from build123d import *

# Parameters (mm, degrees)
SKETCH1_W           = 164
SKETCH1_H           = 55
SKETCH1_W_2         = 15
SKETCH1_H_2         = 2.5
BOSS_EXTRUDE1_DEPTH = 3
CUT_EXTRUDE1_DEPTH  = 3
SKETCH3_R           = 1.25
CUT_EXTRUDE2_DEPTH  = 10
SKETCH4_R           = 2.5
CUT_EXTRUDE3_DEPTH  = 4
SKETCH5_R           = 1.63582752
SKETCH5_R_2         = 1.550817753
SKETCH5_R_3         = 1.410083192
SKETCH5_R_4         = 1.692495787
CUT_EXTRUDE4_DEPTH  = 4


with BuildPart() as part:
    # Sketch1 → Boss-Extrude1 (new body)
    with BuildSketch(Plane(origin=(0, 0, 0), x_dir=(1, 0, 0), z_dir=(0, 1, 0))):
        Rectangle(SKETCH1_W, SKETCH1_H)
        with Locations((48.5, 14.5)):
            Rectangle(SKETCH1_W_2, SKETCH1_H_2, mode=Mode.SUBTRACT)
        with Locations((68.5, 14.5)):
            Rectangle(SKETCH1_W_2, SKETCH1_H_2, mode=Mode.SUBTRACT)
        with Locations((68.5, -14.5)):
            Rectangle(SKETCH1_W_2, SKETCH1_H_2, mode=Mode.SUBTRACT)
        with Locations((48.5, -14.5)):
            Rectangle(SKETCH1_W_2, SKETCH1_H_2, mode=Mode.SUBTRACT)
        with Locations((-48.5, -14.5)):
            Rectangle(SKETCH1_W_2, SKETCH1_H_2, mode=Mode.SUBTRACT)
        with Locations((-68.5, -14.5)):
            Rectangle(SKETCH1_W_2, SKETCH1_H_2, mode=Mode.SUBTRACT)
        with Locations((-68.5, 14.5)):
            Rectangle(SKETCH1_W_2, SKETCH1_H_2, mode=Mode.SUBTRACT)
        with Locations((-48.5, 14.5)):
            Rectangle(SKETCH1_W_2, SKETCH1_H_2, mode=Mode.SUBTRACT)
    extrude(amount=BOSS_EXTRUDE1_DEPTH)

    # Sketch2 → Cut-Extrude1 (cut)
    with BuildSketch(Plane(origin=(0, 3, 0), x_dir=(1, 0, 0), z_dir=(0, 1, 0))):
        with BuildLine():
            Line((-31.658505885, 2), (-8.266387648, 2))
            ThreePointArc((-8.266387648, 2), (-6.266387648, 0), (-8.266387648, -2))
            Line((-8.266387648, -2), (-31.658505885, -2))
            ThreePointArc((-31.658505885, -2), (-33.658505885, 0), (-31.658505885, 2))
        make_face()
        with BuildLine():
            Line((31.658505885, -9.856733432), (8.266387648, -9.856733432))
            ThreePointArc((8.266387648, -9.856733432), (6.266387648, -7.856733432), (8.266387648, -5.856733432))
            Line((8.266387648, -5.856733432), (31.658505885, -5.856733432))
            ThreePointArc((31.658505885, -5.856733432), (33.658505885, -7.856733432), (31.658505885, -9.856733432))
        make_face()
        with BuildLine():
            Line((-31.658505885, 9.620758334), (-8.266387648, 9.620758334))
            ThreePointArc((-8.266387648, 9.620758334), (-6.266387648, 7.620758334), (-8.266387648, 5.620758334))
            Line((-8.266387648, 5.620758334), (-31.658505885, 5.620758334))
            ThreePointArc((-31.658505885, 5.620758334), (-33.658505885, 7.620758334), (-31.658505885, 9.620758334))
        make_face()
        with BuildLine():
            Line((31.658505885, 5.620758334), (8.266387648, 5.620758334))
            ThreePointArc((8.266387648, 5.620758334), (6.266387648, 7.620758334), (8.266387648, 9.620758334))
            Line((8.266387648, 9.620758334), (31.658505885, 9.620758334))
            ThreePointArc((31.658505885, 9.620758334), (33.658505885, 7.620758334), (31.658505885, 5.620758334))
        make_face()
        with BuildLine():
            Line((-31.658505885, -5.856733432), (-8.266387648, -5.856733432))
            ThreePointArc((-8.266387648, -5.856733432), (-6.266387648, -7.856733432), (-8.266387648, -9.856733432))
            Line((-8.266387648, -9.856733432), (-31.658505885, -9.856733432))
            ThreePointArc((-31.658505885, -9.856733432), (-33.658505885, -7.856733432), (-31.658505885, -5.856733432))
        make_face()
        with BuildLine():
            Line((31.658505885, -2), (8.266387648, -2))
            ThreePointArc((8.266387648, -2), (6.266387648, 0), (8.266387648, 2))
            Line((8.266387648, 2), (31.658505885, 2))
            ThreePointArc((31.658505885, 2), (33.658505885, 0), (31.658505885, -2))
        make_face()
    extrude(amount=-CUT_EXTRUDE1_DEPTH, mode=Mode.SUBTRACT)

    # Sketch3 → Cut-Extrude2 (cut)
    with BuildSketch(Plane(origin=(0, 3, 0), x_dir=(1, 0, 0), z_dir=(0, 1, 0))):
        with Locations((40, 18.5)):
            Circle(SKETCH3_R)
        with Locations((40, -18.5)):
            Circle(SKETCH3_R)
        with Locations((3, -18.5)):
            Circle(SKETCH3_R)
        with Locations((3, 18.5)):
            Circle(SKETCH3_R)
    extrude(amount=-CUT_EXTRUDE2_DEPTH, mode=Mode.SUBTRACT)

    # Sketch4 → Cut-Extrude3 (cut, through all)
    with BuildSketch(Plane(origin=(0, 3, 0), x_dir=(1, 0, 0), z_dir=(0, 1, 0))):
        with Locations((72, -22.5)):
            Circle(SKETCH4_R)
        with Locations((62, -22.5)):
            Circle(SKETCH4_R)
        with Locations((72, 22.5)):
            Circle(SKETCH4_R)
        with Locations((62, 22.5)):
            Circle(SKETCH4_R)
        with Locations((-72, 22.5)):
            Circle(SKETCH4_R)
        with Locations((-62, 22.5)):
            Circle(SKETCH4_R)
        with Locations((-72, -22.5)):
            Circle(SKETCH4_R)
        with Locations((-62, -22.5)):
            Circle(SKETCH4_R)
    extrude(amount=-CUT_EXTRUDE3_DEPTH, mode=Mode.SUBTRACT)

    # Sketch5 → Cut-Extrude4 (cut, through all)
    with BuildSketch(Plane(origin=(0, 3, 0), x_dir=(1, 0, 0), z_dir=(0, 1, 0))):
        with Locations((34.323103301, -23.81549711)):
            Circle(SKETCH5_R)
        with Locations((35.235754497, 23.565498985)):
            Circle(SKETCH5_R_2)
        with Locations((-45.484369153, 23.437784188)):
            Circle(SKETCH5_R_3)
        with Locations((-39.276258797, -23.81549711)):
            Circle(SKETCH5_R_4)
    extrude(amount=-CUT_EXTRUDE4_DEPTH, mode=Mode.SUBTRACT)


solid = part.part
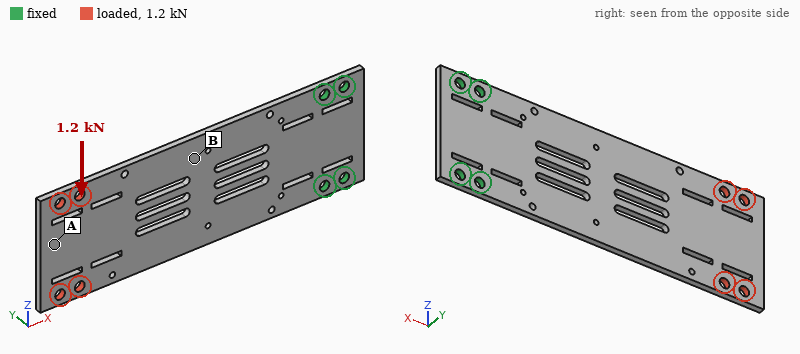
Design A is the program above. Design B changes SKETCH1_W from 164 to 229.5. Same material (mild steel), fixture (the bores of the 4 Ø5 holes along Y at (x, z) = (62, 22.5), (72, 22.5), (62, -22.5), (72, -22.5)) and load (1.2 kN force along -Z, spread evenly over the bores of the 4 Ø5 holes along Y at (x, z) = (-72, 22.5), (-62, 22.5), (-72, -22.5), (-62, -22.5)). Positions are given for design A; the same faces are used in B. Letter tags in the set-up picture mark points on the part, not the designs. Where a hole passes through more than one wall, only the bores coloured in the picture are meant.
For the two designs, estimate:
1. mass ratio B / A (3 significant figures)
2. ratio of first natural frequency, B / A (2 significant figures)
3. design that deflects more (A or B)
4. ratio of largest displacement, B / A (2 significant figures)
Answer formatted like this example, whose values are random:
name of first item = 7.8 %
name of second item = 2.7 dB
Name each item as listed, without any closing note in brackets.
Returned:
mass ratio B / A = 1.46
ratio of first natural frequency, B / A = 0.64
design that deflects more = B
ratio of largest displacement, B / A = 1.2
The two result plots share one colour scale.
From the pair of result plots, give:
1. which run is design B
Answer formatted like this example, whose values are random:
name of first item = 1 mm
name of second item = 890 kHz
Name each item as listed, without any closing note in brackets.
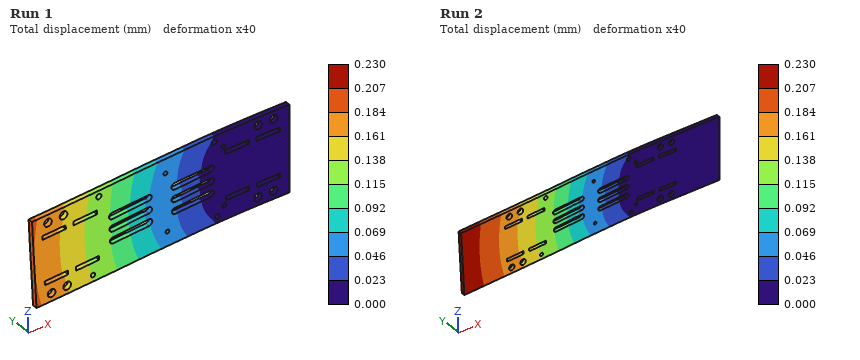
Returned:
which run is design B = Run 2
